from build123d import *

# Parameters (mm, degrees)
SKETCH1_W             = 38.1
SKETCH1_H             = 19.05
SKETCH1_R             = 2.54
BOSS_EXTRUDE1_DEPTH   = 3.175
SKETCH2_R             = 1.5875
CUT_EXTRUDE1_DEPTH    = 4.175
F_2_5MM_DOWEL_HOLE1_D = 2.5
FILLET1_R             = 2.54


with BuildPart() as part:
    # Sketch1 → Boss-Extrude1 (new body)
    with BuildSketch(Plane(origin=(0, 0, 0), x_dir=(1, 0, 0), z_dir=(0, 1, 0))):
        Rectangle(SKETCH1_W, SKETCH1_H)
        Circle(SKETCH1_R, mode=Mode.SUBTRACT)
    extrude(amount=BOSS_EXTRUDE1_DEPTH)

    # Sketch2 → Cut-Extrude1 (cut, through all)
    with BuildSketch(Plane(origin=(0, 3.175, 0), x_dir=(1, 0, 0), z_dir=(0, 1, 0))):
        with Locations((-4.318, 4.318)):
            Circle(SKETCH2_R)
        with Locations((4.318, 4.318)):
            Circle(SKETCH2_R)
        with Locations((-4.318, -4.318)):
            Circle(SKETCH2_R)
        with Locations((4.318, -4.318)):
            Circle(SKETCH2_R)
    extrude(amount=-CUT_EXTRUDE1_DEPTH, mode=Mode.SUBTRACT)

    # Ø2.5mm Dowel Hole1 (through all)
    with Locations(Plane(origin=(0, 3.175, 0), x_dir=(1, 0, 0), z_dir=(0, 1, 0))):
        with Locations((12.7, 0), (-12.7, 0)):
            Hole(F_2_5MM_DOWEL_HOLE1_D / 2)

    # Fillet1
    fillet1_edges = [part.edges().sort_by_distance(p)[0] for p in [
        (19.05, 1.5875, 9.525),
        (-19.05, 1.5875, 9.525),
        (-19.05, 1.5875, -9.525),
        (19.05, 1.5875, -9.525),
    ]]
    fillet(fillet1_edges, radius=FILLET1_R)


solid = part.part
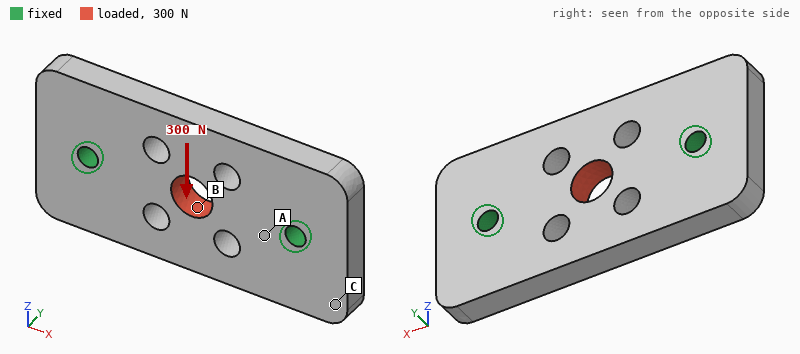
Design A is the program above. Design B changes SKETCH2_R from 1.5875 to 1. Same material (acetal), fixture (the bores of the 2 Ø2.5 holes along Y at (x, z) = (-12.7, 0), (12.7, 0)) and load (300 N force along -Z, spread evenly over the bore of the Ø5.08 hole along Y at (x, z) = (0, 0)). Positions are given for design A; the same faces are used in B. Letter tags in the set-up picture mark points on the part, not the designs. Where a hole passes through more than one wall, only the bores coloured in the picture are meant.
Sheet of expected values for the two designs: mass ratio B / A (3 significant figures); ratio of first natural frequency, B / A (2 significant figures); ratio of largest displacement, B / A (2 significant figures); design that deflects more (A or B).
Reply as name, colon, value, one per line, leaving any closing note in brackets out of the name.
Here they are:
mass ratio B / A: 1.03
ratio of first natural frequency, B / A: 1.00
ratio of largest displacement, B / A: 0.87
design that deflects more: A
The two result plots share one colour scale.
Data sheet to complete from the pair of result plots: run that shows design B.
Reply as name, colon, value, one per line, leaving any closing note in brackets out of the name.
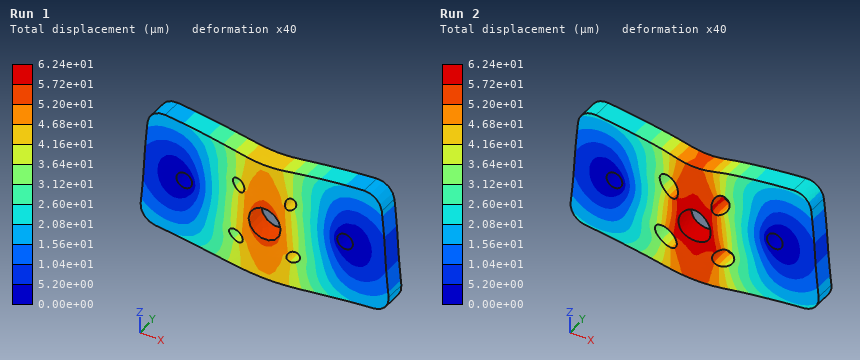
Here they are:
run that shows design B: Run 1
